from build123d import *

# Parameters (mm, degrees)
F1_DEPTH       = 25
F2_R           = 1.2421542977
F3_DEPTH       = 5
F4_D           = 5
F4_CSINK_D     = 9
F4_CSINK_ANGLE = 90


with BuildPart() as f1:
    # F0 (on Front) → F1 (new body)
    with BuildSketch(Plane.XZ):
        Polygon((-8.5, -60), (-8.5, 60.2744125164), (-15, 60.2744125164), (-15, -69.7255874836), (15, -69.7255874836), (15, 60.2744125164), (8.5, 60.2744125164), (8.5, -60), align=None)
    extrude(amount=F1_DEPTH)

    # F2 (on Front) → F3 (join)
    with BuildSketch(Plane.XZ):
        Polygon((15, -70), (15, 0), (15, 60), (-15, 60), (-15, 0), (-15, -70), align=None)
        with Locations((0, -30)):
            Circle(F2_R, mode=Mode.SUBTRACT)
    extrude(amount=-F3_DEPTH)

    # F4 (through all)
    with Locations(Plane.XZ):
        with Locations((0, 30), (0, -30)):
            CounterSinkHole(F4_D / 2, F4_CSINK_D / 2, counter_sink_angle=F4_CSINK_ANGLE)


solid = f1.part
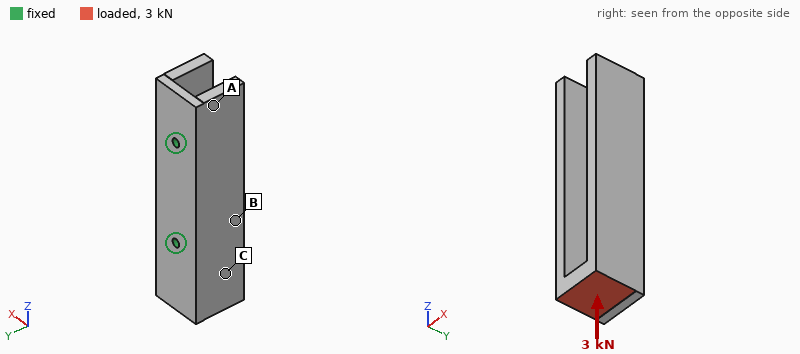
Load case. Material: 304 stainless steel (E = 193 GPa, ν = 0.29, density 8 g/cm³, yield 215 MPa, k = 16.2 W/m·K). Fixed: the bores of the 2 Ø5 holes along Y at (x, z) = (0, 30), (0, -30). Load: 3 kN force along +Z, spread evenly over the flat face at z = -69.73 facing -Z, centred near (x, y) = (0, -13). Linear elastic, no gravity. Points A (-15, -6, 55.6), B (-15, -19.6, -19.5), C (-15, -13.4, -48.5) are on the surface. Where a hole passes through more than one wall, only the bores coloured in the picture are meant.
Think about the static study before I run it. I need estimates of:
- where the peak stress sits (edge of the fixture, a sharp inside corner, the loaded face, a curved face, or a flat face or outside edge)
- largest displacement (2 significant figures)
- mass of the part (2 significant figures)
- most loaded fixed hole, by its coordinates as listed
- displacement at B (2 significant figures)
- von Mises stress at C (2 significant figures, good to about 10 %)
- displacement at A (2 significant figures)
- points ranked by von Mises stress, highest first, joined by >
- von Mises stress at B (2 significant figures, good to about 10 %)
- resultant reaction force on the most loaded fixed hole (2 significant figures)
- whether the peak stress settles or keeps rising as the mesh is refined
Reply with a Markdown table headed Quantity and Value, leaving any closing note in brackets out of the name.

| Quantity | Value |
|---|---|
| where the peak stress sits | edge of the fixture |
| largest displacement | 13 µm |
| mass of the part | 520 g |
| most loaded fixed hole, by its coordinates as listed | (0, -30) |
| displacement at B | 3.9 µm |
| von Mises stress at C | 6.6 MPa |
| displacement at A | 5.6 µm |
| points ranked by von Mises stress, highest first, joined by > | B > C > A |
| von Mises stress at B | 12 MPa |
| resultant reaction force on the most loaded fixed hole | 1.8 kN |
| whether the peak stress settles or keeps rising as the mesh is refined | keeps rising |
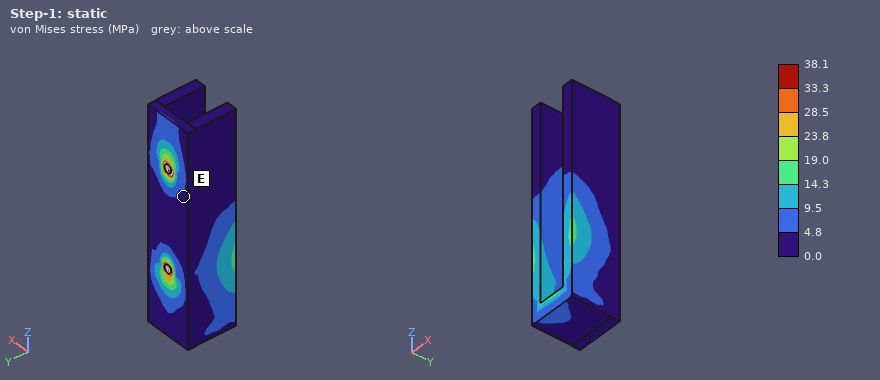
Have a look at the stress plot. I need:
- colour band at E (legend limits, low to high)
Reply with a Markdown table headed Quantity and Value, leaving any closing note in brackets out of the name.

| Quantity | Value |
|---|---|
| colour band at E | 0.0 to 4.8 MPa |
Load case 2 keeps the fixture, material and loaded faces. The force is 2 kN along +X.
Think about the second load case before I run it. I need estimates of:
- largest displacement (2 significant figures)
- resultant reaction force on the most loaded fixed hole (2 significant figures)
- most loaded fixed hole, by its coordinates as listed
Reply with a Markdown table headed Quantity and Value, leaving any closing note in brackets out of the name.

| Quantity | Value |
|---|---|
| largest displacement | 0.12 mm |
| resultant reaction force on the most loaded fixed hole | 3.2 kN |
| most loaded fixed hole, by its coordinates as listed | (0, -30) |
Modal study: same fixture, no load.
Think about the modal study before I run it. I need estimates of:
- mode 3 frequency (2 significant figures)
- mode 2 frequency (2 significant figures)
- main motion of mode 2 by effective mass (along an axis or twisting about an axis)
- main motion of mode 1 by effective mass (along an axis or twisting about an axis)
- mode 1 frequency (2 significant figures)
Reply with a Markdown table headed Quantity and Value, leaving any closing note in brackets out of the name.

| Quantity | Value |
|---|---|
| mode 3 frequency | 3400 Hz |
| mode 2 frequency | 2800 Hz |
| main motion of mode 2 by effective mass | twisting about Y |
| main motion of mode 1 by effective mass | along X |
| mode 1 frequency | 1500 Hz |
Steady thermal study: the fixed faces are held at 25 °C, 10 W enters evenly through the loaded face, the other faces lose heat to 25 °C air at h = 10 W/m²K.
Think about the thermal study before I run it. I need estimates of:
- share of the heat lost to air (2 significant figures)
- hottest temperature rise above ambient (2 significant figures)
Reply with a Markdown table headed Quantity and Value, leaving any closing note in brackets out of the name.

| Quantity | Value |
|---|---|
| share of the heat lost to air | 39 % |
| hottest temperature rise above ambient | 62 K |
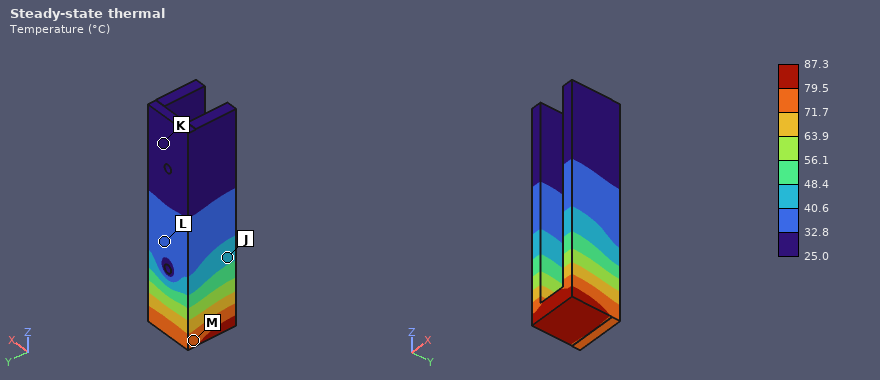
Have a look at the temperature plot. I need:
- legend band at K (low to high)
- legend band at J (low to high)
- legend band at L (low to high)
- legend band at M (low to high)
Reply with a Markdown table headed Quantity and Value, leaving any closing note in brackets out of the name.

| Quantity | Value |
|---|---|
| legend band at K | 25.0 to 32.8 °C |
| legend band at J | 40.6 to 48.4 °C |
| legend band at L | 32.8 to 40.6 °C |
| legend band at M | 71.7 to 79.5 °C |
